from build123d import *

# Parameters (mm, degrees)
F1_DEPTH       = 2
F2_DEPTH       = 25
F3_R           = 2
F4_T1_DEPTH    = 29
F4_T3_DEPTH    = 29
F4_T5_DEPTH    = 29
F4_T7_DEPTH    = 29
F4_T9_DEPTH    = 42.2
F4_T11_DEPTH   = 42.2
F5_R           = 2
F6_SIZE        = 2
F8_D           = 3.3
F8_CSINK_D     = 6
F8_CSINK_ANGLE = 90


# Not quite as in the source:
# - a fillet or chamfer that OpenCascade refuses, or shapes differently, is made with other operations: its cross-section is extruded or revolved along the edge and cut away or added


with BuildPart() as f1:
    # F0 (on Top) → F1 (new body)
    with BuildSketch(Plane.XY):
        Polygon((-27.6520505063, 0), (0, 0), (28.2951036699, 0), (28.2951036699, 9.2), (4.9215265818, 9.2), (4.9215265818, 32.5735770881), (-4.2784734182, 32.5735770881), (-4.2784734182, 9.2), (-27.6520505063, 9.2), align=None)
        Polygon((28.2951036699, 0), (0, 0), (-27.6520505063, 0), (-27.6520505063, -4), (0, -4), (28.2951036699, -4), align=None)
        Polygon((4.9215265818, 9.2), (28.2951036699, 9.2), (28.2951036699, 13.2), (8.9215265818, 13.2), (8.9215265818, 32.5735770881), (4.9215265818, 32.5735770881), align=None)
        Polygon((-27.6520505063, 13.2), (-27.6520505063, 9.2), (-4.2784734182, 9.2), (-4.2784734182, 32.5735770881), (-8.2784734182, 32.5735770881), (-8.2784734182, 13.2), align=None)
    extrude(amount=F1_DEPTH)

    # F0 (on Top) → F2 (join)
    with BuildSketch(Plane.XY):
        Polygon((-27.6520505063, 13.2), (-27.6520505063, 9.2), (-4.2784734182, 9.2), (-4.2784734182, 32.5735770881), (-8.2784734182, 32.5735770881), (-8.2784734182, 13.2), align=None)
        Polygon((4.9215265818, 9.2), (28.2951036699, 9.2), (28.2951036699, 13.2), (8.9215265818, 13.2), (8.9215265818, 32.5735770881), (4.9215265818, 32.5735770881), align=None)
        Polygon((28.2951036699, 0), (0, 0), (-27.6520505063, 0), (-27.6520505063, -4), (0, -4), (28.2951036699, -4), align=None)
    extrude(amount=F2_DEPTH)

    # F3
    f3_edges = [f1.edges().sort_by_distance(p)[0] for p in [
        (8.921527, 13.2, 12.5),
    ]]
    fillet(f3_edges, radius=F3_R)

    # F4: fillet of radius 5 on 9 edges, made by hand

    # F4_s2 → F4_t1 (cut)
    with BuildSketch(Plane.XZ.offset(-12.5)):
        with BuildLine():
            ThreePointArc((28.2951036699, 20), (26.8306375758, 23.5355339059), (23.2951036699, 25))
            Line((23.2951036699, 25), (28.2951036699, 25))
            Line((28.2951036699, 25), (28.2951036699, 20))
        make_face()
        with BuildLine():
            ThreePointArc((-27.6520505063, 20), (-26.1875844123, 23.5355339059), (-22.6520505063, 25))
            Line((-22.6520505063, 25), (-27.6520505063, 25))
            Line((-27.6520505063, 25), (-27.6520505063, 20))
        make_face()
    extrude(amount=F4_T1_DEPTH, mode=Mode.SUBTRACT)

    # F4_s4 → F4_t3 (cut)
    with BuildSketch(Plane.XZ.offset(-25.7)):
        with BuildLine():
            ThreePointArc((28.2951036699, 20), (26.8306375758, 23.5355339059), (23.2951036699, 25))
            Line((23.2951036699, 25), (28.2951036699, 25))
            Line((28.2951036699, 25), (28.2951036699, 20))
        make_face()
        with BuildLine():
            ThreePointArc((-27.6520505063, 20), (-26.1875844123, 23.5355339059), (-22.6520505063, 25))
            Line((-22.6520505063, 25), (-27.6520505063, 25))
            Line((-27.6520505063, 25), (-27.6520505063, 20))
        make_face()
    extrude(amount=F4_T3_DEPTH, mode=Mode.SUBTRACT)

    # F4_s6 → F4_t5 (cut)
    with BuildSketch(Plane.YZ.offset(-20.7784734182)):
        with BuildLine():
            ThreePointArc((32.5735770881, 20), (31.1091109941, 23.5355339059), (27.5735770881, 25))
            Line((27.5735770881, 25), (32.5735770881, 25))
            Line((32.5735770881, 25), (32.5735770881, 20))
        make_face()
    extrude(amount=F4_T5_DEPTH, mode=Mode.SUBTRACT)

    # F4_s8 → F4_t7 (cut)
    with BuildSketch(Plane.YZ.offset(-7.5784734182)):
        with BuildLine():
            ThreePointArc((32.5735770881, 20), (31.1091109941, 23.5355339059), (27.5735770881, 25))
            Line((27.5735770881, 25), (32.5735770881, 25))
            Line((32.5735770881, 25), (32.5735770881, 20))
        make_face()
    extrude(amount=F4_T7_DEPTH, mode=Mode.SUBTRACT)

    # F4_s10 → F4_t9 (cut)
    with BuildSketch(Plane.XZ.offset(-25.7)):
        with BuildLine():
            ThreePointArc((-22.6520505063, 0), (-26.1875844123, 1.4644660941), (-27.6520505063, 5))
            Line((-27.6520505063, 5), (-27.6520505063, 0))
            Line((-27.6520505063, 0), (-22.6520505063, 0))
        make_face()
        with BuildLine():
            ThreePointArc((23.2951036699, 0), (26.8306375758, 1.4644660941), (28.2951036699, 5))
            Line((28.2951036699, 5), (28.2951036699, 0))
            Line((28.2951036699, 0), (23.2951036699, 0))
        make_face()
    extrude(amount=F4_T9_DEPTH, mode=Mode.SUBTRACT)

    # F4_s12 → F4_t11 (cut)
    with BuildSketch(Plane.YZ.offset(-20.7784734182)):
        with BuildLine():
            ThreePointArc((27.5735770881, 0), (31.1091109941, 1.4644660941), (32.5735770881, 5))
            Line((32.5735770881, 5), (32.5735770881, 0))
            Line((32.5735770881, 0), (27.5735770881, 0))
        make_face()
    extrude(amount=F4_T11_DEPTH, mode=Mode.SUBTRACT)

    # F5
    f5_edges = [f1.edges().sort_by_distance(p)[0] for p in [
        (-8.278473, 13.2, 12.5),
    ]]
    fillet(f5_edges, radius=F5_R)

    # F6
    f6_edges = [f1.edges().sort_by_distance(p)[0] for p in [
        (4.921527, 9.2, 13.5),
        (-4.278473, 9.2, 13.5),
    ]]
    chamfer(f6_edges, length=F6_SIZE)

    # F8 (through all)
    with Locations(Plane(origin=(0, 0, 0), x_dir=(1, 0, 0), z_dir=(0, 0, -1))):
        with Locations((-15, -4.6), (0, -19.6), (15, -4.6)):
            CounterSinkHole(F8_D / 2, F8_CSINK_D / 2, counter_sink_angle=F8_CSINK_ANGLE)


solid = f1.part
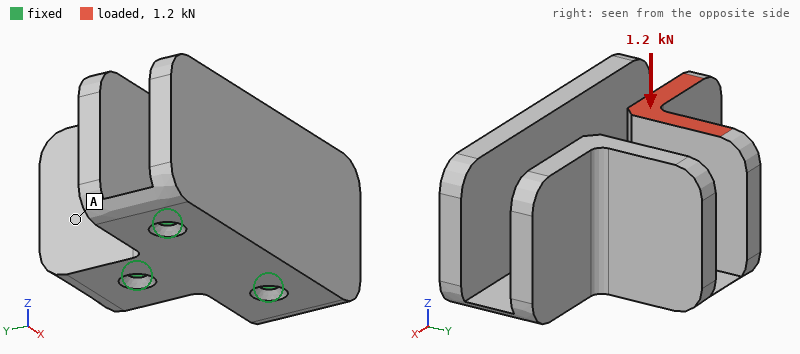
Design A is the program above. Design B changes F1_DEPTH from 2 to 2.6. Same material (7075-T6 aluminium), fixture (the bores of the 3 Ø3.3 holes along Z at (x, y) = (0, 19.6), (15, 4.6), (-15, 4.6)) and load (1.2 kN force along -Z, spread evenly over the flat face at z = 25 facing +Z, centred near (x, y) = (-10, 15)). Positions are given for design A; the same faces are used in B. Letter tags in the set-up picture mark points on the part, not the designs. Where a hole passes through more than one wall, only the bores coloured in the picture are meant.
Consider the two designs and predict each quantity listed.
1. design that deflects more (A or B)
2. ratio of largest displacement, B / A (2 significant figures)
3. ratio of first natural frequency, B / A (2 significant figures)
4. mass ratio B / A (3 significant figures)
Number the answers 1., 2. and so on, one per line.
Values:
1. A
2. 0.50
3. 1.5
4. 1.03
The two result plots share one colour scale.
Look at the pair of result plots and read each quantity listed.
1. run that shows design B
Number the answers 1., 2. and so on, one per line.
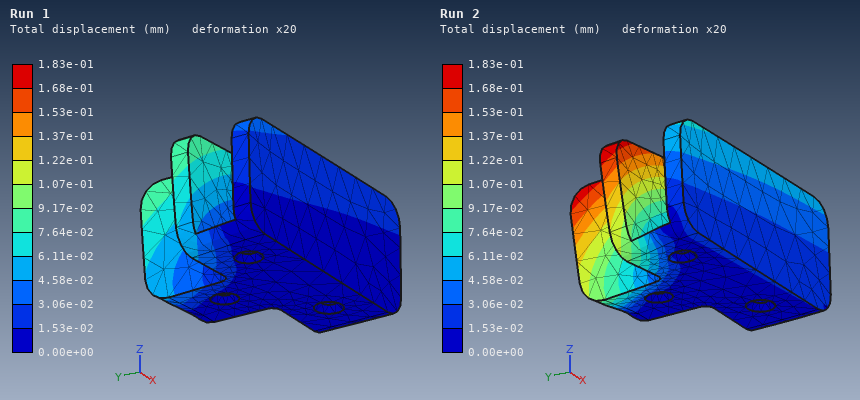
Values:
1. Run 1
